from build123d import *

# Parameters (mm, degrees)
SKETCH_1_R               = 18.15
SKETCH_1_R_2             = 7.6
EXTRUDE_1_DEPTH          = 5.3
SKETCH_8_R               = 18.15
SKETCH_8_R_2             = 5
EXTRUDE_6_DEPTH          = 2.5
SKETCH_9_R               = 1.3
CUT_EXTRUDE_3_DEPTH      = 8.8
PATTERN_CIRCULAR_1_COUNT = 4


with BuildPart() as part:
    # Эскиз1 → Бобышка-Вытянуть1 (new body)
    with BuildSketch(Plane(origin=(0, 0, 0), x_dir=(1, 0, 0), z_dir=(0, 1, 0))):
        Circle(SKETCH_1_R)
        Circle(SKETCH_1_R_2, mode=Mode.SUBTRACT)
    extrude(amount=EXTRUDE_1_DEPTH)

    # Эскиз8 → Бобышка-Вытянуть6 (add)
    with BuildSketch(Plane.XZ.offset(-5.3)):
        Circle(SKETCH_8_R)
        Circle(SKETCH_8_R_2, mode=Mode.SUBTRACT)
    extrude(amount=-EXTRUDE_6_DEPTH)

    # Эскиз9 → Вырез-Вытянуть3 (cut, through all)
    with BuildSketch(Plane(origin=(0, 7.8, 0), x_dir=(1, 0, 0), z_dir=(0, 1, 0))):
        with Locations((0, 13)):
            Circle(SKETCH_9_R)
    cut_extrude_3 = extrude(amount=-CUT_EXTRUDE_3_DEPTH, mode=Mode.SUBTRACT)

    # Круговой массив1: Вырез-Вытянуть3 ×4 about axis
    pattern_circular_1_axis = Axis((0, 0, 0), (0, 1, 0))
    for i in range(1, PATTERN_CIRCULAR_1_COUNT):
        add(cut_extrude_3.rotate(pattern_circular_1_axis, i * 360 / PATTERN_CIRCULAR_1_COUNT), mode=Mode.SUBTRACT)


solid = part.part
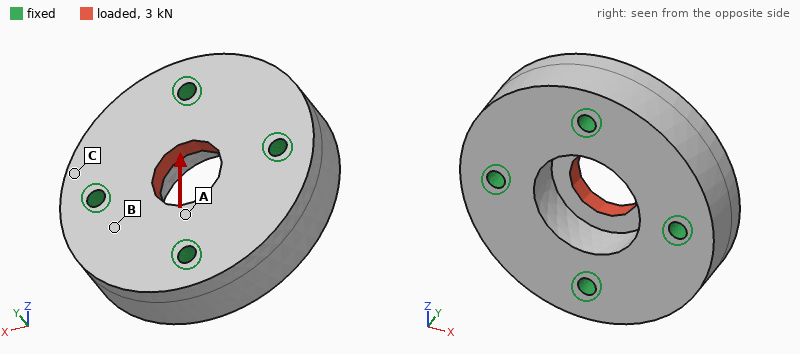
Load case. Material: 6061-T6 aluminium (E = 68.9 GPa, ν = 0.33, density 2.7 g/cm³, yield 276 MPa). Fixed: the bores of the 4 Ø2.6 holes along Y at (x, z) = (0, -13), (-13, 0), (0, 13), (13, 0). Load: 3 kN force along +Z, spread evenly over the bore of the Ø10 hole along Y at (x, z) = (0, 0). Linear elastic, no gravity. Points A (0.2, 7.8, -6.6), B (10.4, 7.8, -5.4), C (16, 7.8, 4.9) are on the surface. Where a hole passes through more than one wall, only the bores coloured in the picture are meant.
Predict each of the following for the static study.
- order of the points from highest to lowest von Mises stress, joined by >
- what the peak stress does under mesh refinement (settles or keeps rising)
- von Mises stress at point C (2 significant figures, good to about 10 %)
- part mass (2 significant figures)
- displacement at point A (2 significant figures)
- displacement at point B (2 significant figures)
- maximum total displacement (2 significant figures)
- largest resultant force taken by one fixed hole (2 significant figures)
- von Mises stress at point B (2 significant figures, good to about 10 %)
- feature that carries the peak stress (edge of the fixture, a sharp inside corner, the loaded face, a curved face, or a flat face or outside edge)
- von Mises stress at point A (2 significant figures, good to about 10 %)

A > B > C
keeps rising
5.4 MPa
18 g
3.9 µm
1.5 µm
5.2 µm
900 N
11 MPa
edge of the fixture
44 MPa
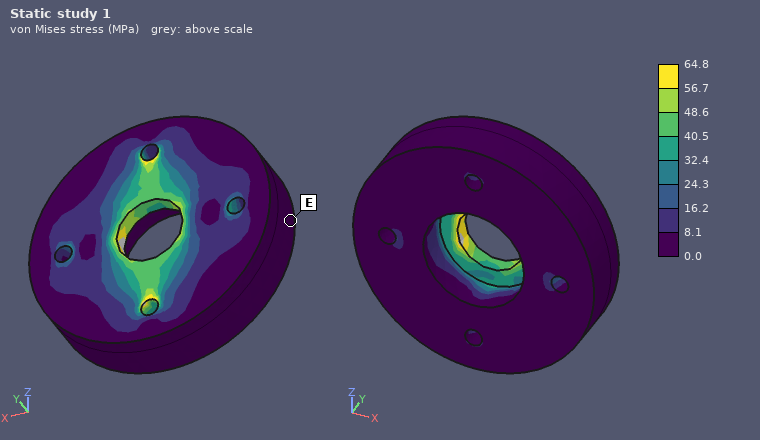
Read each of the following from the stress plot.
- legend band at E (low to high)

0.0 to 8.1 MPa
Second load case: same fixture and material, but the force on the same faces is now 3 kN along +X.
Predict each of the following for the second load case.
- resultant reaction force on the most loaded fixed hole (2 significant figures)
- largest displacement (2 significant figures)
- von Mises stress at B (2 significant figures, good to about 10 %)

900 N
5.2 µm
14 MPa
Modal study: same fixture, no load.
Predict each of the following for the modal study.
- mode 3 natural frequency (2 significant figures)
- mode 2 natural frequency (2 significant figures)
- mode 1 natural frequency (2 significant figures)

47 kHz
47 kHz
44 kHz
